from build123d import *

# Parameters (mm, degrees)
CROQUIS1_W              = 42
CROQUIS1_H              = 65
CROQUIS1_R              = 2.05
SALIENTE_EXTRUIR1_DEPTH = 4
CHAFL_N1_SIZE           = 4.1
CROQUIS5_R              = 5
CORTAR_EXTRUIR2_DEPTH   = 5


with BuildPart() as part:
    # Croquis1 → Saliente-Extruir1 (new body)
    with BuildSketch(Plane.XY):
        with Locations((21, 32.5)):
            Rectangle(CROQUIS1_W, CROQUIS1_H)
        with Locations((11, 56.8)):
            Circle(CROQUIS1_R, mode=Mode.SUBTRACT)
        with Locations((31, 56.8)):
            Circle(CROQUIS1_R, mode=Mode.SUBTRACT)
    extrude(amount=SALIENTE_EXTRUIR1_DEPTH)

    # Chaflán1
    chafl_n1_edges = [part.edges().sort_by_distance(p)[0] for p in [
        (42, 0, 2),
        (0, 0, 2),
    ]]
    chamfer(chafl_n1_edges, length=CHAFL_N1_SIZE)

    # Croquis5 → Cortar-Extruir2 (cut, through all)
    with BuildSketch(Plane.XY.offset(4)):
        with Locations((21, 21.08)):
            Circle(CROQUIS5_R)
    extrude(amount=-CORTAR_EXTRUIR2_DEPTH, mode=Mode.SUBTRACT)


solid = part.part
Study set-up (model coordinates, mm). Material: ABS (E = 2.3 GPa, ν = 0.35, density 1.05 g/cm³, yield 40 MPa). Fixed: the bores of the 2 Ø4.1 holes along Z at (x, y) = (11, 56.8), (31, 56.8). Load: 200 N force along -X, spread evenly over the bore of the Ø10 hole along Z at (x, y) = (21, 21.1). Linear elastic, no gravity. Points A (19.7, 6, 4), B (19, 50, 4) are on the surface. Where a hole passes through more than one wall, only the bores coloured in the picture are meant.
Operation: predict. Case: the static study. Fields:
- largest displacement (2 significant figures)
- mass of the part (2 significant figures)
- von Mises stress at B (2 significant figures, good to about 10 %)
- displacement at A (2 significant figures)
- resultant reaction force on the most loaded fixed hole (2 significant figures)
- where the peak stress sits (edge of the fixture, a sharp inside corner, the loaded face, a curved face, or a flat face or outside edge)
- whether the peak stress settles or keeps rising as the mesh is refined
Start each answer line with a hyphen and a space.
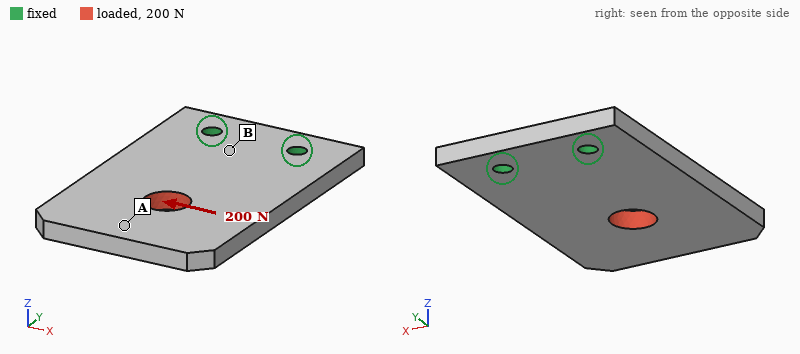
- 0.26 mm
- 11 g
- 4.4 MPa
- 0.23 mm
- 330 N
- edge of the fixture
- keeps rising
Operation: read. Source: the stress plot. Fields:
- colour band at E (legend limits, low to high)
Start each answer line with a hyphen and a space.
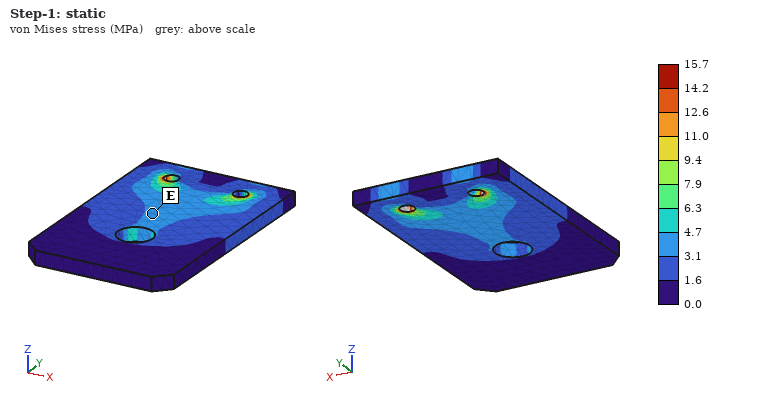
- 3.1 to 4.7 MPa
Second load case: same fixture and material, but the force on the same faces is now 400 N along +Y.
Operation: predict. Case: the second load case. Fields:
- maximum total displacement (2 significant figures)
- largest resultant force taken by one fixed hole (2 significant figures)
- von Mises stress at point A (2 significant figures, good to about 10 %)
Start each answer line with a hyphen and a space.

- 64 µm
- 200 N
- 1.3 MPa
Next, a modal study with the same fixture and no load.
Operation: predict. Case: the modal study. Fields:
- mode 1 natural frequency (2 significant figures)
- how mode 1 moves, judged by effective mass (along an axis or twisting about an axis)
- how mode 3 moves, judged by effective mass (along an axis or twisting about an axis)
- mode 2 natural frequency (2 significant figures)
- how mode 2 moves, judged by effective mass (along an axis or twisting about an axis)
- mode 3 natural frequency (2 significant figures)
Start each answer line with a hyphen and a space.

- 310 Hz
- along Z
- along Z
- 870 Hz
- twisting about Y
- 1800 Hz
